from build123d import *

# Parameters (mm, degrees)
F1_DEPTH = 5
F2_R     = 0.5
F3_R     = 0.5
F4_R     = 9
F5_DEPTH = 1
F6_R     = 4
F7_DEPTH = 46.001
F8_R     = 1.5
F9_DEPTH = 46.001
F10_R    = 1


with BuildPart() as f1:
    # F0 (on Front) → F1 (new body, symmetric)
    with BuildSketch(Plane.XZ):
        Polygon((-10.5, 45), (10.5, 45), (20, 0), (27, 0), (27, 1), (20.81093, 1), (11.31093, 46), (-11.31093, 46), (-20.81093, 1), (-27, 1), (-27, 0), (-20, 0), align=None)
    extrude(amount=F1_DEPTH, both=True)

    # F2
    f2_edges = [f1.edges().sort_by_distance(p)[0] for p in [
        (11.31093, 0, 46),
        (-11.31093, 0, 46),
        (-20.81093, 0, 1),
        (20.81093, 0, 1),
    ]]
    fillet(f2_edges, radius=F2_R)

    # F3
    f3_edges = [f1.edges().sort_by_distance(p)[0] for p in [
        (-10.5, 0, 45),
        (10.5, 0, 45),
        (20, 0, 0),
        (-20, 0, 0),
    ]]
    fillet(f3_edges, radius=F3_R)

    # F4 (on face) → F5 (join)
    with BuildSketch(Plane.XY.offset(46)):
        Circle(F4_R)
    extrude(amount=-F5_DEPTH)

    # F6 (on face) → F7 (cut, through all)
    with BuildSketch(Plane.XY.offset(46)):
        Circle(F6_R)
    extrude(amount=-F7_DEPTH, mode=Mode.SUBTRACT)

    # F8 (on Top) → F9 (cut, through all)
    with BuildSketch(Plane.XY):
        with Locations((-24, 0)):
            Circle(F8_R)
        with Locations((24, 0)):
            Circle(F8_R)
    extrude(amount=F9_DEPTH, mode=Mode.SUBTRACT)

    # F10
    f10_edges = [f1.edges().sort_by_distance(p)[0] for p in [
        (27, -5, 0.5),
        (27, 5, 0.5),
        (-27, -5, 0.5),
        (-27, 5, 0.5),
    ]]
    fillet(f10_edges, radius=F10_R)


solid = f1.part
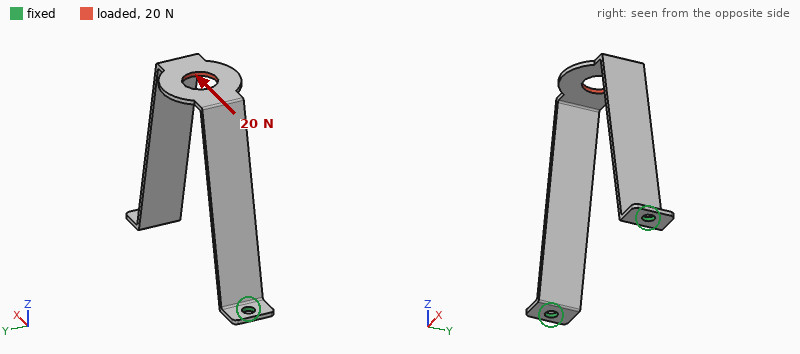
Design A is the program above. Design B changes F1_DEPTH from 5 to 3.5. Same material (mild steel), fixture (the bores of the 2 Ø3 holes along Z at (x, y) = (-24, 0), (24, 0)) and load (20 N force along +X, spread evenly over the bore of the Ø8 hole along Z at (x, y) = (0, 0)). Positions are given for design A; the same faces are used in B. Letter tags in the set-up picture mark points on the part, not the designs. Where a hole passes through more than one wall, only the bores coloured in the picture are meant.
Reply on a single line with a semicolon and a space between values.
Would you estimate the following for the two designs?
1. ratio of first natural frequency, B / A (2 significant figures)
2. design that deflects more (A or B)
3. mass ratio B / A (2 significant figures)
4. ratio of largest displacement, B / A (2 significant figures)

0.95; B; 0.74; 1.4
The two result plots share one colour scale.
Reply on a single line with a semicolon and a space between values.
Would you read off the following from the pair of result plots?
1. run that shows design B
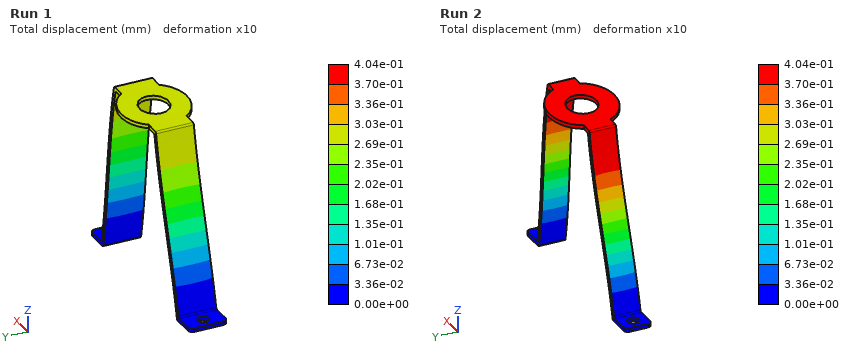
Run 2
